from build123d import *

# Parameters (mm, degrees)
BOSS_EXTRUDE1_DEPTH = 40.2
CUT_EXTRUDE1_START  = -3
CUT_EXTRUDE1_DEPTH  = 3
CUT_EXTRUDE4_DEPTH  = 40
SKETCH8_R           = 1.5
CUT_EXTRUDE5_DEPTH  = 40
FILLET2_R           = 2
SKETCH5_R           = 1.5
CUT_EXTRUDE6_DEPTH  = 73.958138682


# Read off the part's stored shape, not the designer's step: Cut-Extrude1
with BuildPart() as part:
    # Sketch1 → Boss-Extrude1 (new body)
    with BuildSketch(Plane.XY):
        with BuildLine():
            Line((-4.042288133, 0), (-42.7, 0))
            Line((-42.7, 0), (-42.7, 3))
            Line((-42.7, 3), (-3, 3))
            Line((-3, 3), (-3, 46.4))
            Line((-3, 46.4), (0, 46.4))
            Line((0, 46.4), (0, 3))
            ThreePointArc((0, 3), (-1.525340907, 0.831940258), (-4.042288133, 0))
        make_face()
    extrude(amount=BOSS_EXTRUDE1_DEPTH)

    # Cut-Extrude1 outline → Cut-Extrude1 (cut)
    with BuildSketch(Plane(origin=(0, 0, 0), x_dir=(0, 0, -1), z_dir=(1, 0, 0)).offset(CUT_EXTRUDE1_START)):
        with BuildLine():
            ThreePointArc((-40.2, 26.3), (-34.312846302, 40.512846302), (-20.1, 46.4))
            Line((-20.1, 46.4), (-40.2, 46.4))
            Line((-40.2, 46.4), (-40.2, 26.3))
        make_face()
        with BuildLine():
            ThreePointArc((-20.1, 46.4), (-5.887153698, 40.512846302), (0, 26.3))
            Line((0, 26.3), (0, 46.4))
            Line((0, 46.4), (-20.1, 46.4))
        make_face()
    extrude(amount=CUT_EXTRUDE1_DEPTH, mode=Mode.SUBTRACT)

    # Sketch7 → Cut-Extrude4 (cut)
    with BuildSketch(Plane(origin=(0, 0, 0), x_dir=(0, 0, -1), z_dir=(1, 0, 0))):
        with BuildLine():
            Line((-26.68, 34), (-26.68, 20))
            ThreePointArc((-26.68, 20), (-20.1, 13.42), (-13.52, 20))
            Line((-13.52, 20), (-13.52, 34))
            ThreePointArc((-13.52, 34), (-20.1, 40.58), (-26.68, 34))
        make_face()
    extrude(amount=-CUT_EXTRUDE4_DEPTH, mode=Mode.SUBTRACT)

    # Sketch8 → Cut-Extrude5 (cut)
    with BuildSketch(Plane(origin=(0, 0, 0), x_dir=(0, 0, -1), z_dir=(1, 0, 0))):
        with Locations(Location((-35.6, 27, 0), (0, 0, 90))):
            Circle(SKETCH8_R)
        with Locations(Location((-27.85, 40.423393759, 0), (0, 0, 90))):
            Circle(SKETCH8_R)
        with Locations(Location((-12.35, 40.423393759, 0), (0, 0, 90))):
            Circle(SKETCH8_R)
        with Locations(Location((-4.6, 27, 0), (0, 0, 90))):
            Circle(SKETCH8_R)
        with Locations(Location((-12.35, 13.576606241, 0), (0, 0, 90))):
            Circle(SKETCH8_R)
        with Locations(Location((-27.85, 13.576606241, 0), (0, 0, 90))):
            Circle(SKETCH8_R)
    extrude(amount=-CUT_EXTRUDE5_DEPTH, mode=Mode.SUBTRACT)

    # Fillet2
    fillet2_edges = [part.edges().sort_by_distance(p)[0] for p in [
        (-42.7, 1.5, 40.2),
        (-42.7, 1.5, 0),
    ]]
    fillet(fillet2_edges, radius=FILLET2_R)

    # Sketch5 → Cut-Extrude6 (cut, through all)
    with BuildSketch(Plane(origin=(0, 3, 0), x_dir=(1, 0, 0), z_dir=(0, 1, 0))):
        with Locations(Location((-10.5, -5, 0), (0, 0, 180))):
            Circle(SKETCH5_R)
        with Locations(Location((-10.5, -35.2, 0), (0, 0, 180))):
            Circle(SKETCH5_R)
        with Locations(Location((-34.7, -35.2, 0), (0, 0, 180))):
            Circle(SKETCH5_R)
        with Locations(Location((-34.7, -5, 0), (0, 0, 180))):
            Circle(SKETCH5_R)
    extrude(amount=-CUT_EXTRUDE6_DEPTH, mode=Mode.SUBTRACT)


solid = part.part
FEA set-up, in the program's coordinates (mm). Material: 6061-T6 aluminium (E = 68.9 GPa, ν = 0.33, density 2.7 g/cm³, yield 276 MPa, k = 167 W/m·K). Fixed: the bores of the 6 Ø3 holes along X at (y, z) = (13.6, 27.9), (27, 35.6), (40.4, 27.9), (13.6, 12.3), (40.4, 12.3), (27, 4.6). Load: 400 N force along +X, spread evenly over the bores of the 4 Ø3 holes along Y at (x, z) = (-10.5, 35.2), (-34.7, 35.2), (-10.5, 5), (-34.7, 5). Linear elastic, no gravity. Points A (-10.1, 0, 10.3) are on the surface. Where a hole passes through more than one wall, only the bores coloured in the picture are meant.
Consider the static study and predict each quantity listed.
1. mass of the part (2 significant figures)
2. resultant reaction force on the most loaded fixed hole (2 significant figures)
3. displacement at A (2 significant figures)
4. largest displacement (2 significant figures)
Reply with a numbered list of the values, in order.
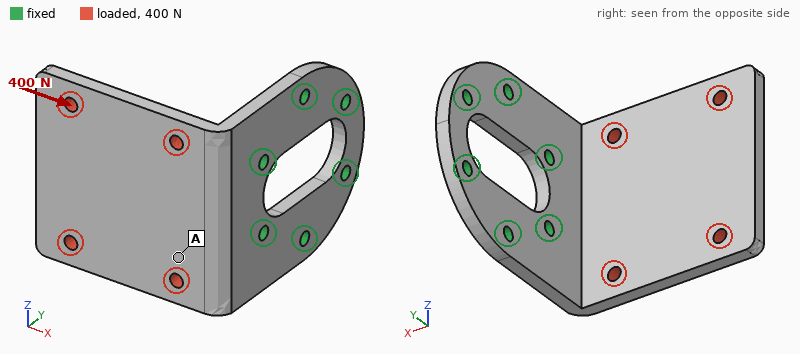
1. 23 g
2. 250 N
3. 0.069 mm
4. 0.22 mm
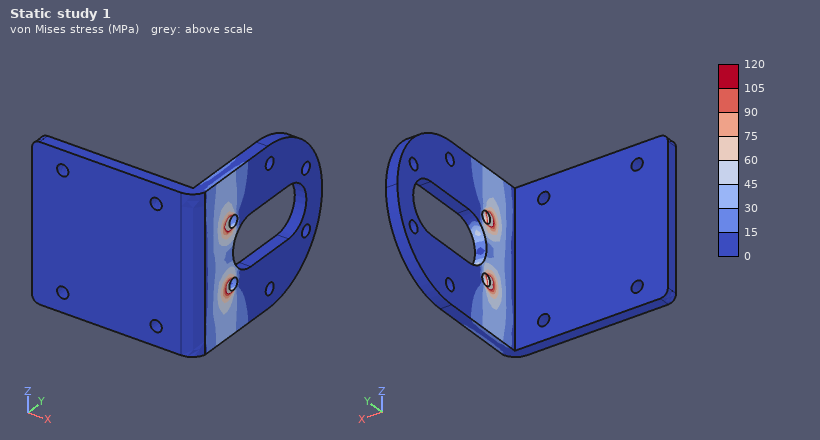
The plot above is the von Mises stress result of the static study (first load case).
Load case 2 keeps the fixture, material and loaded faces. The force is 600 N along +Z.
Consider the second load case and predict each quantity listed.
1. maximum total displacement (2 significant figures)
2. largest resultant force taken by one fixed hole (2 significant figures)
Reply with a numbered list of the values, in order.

1. 0.31 mm
2. 720 N
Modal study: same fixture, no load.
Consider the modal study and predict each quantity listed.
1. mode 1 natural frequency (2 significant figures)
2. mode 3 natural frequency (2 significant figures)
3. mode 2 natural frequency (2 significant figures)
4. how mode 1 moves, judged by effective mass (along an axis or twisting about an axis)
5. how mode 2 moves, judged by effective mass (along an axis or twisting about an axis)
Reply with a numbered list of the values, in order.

1. 990 Hz
2. 3500 Hz
3. 2200 Hz
4. along Y
5. along Z
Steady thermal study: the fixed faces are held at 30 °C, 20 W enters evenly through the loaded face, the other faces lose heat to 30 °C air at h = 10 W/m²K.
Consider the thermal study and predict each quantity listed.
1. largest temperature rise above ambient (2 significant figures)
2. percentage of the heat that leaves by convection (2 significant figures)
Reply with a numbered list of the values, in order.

1. 36 K
2. 5.2 %
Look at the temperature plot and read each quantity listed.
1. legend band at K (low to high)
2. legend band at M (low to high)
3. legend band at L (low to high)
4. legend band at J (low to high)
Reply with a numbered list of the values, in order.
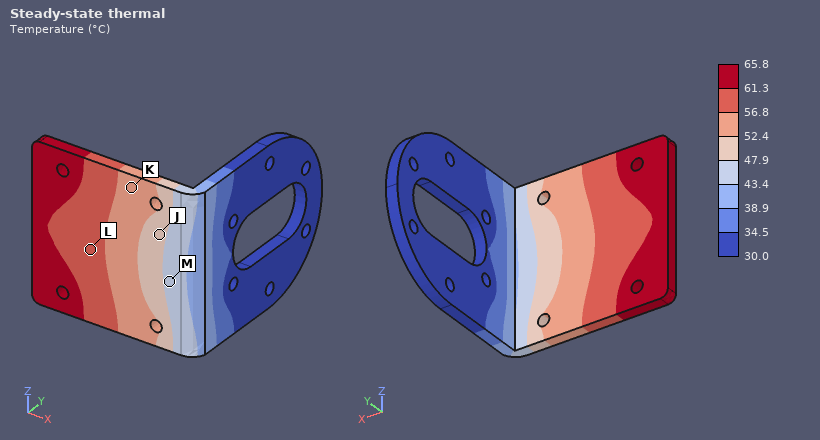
1. 52.4 to 56.8 °C
2. 43.4 to 47.9 °C
3. 56.8 to 61.3 °C
4. 47.9 to 52.4 °C
